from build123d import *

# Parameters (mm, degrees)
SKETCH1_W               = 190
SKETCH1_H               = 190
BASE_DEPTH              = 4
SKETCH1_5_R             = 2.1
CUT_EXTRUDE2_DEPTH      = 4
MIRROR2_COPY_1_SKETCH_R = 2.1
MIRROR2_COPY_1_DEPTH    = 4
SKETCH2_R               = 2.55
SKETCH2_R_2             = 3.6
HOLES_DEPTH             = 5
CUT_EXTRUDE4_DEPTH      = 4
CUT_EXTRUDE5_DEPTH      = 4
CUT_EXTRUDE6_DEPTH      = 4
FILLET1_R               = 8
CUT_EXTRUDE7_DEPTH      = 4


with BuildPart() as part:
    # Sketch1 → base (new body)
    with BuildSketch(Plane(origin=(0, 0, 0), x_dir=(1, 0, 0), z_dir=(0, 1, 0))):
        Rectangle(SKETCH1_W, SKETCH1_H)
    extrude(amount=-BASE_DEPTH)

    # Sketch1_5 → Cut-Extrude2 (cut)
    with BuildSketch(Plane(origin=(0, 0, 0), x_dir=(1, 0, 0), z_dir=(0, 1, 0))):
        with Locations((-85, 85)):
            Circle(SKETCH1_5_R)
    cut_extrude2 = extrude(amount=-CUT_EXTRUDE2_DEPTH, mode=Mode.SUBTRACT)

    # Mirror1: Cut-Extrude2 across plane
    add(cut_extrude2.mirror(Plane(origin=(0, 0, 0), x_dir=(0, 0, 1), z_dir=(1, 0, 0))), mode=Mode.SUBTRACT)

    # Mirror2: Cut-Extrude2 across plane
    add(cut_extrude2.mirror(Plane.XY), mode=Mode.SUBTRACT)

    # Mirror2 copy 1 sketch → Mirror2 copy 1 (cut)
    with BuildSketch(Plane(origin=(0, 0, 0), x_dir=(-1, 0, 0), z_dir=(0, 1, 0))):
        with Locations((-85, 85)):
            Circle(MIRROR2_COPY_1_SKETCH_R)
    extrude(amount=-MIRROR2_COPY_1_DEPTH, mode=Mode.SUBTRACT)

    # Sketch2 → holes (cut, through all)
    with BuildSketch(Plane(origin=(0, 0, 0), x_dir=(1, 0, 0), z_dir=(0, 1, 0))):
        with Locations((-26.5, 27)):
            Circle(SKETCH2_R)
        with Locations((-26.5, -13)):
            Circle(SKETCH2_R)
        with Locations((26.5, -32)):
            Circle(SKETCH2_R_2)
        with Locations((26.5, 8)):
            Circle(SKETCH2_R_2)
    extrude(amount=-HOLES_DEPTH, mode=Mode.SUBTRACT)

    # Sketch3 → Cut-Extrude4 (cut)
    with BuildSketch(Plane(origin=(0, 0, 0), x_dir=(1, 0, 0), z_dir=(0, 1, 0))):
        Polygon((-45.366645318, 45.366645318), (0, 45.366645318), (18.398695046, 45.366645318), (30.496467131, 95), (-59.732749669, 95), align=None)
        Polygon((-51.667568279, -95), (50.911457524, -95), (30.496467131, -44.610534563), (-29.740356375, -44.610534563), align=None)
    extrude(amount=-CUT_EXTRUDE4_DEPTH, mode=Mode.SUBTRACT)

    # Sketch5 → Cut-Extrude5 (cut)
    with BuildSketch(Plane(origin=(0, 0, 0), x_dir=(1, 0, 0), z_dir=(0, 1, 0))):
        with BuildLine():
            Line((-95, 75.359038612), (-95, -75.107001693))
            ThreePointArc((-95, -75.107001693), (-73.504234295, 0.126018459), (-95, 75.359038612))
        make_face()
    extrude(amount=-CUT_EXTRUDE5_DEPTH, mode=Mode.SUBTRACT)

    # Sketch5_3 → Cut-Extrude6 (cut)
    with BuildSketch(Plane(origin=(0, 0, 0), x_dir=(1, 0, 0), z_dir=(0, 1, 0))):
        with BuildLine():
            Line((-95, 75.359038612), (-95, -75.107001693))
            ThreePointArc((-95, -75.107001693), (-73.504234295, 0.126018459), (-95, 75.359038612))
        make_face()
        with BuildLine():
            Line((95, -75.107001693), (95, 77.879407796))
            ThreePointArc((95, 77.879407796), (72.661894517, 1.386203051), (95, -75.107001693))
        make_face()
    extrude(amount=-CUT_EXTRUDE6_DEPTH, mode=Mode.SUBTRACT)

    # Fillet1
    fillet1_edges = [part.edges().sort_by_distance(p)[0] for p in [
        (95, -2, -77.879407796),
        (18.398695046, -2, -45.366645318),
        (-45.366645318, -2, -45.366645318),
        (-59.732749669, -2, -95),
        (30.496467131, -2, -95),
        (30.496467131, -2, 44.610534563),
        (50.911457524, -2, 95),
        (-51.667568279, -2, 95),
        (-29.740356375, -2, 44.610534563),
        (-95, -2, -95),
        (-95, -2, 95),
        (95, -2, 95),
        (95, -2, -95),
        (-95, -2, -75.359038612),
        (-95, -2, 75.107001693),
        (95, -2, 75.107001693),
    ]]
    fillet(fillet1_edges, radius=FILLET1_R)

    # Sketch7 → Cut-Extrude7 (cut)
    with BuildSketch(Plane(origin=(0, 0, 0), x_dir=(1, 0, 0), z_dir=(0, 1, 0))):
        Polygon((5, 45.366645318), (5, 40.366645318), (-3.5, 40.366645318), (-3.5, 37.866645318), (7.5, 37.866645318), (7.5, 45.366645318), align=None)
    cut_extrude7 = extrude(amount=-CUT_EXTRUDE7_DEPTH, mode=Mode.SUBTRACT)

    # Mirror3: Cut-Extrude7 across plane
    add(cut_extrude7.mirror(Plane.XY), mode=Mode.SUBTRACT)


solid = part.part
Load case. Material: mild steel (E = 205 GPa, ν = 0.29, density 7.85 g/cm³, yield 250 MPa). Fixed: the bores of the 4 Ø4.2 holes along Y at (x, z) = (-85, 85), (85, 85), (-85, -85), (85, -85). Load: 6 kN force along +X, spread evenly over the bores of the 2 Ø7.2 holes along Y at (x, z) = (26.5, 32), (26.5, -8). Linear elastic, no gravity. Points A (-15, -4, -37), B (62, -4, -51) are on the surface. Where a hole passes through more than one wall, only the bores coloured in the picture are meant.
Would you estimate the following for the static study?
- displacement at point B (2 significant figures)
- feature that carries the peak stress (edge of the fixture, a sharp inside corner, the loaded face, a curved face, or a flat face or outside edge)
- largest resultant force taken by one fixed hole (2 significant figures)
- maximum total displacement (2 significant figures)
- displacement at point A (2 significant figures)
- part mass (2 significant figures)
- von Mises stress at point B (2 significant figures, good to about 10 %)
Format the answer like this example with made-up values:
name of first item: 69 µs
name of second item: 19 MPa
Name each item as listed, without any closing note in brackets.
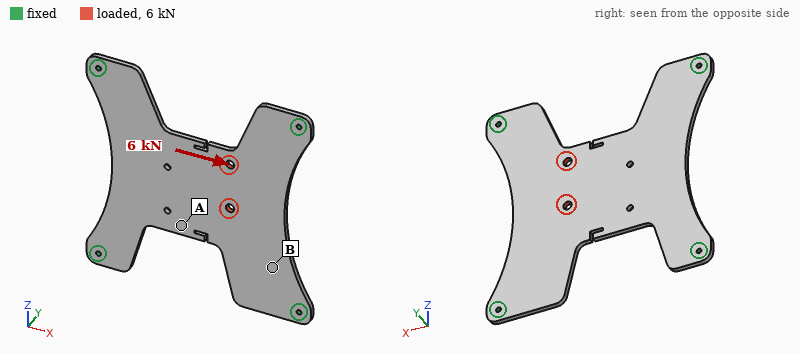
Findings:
displacement at point B: 6.3 µm
feature that carries the peak stress: edge of the fixture
largest resultant force taken by one fixed hole: 2.5 kN
maximum total displacement: 15 µm
displacement at point A: 10 µm
part mass: 730 g
von Mises stress at point B: 14 MPa
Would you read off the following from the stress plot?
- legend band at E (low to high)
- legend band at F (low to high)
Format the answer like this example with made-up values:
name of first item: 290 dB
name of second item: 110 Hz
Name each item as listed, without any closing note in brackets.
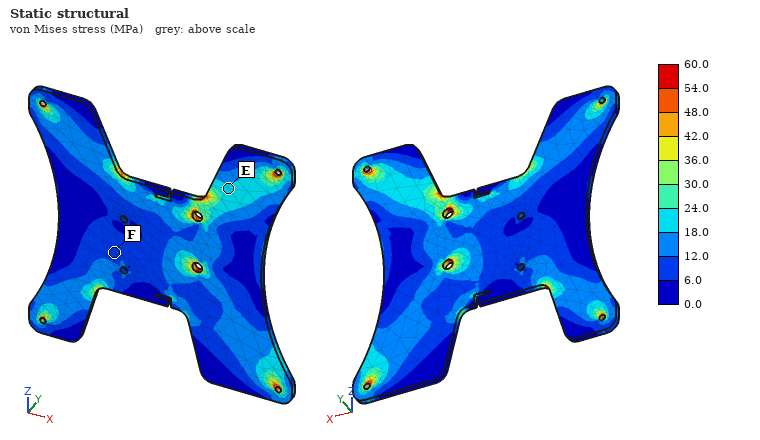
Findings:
legend band at E: 18.0 to 24.0 MPa
legend band at F: 6.0 to 12.0 MPa
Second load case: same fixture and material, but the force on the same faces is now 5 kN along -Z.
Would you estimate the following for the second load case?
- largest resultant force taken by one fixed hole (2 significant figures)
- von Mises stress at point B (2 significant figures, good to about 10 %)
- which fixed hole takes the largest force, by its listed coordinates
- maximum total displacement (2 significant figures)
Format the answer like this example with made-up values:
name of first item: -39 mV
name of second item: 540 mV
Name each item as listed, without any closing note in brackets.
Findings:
largest resultant force taken by one fixed hole: 2.3 kN
von Mises stress at point B: 13 MPa
which fixed hole takes the largest force, by its listed coordinates: (85, 85)
maximum total displacement: 11 µm
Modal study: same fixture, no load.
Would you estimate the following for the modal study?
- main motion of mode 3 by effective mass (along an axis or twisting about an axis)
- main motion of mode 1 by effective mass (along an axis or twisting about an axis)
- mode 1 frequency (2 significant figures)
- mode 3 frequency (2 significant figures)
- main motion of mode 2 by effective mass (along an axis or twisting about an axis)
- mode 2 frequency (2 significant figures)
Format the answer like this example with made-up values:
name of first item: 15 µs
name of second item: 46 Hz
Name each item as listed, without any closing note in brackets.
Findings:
main motion of mode 3 by effective mass: twisting about X
main motion of mode 1 by effective mass: along Y
mode 1 frequency: 410 Hz
mode 3 frequency: 980 Hz
main motion of mode 2 by effective mass: twisting about Z
mode 2 frequency: 800 Hz
